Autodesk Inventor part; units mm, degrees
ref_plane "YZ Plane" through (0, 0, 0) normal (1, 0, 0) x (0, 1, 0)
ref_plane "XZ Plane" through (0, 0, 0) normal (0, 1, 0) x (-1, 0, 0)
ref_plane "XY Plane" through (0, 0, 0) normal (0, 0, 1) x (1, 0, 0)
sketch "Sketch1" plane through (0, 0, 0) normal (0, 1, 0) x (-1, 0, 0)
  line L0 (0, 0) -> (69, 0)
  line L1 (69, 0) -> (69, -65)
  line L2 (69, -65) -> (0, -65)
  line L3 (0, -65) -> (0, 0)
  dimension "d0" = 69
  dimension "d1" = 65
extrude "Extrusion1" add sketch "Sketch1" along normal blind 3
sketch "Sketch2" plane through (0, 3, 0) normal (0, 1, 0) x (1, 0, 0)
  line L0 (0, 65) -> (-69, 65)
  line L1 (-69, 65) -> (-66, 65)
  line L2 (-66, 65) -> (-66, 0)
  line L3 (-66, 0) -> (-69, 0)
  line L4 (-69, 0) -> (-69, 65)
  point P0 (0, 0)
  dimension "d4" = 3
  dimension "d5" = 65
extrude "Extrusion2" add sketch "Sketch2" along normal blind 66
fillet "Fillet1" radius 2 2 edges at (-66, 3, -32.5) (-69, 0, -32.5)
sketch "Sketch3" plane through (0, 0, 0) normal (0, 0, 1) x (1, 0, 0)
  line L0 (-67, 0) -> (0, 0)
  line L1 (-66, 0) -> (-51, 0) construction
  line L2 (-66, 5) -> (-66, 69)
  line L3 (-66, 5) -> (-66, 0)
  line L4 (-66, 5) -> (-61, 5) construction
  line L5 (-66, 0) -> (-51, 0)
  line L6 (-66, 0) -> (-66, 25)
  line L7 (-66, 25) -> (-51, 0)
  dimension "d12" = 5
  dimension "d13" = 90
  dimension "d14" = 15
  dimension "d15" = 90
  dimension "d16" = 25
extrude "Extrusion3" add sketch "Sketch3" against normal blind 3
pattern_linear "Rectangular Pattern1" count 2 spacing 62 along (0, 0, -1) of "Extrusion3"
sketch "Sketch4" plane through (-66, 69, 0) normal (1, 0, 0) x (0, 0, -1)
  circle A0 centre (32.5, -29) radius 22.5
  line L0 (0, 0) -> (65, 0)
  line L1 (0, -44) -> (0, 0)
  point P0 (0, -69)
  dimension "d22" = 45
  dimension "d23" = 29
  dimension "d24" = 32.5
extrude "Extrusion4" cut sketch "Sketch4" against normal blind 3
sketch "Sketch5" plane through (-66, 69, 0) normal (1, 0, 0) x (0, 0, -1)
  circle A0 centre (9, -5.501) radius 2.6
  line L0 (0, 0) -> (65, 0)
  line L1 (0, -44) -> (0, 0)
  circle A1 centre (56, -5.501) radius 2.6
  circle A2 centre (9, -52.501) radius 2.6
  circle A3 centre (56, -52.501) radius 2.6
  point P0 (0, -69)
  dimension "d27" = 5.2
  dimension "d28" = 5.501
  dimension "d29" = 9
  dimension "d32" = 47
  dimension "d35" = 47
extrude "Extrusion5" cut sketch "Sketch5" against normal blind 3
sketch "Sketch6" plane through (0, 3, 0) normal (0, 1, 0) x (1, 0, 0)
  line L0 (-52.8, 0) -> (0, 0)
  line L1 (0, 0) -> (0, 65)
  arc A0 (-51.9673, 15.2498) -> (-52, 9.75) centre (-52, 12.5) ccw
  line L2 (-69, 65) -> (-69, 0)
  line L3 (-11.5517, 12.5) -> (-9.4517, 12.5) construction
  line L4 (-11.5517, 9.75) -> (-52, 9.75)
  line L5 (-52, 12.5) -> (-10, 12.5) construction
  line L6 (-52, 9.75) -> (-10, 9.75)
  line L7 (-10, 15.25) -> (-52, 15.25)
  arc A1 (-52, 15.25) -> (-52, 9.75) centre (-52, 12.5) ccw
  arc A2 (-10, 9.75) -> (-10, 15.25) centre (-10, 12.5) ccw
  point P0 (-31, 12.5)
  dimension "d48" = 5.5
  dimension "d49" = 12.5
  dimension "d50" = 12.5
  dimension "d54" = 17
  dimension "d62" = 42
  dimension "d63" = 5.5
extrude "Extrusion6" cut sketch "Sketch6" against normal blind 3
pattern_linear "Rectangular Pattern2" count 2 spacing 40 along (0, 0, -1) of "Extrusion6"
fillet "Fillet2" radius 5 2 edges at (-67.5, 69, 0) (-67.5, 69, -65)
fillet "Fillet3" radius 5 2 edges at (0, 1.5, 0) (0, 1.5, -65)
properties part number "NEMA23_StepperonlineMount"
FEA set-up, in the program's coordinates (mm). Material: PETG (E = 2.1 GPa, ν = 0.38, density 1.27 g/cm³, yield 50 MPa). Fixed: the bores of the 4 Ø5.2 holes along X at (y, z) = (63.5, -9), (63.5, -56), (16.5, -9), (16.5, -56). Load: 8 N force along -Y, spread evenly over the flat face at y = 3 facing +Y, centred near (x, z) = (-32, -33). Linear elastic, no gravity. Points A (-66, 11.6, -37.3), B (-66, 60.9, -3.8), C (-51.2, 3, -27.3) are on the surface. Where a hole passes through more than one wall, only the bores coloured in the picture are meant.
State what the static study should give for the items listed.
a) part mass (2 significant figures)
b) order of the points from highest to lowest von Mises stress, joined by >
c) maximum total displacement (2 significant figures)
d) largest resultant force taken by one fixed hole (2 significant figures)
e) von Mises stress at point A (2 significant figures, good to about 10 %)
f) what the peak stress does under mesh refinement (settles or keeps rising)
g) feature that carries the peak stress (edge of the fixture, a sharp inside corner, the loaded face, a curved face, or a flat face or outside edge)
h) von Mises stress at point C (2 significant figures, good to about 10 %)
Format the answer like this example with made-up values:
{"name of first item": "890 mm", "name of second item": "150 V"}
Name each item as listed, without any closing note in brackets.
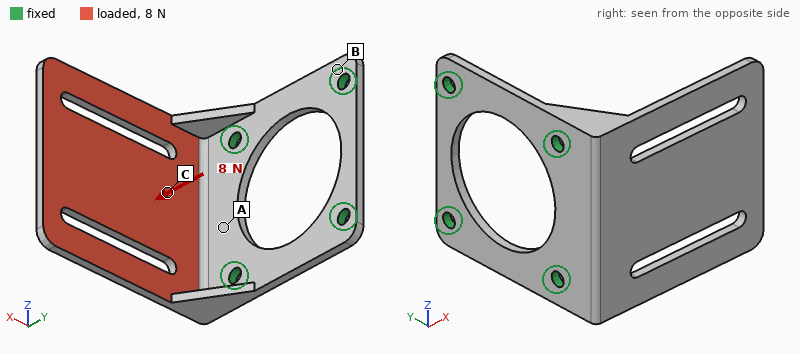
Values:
{"part mass": "26 g", "order of the points from highest to lowest von Mises stress, joined by >": "C > A > B", "maximum total displacement": "1.2 mm", "largest resultant force taken by one fixed hole": "5.1 N", "von Mises stress at point A": "0.83 MPa", "what the peak stress does under mesh refinement": "keeps rising", "feature that carries the peak stress": "edge of the fixture", "von Mises stress at point C": "1.4 MPa"}
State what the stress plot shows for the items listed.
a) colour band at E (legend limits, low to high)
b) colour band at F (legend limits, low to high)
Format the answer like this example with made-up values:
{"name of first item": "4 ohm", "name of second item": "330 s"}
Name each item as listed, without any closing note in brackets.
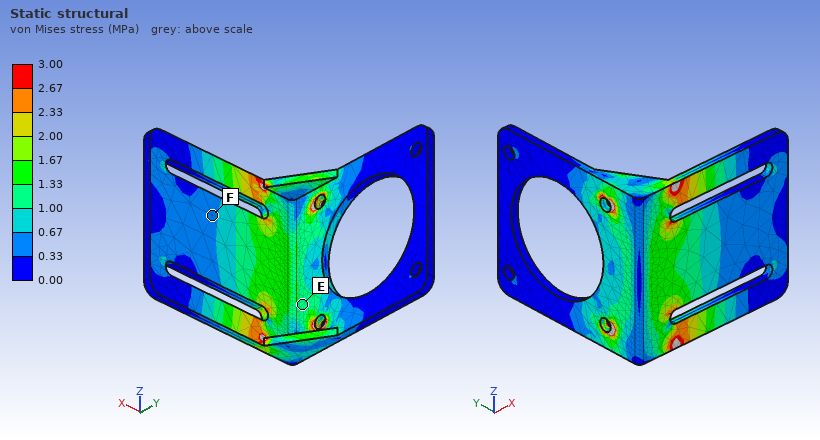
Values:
{"colour band at E": "1.00 to 1.33 MPa", "colour band at F": "0.33 to 0.67 MPa"}
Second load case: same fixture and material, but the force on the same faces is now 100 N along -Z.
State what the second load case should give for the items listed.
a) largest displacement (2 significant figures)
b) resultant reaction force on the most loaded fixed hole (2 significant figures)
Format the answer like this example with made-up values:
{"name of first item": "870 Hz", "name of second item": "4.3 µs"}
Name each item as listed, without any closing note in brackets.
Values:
{"largest displacement": "1.2 mm", "resultant reaction force on the most loaded fixed hole": "92 N"}
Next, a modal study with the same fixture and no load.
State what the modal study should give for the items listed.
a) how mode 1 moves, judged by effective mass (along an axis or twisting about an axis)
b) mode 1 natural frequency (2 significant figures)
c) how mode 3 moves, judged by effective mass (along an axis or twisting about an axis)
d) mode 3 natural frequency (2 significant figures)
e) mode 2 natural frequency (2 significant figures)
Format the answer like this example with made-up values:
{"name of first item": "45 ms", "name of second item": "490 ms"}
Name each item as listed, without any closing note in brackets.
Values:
{"how mode 1 moves, judged by effective mass": "along Y", "mode 1 natural frequency": "140 Hz", "how mode 3 moves, judged by effective mass": "along Z", "mode 3 natural frequency": "560 Hz", "mode 2 natural frequency": "350 Hz"}
